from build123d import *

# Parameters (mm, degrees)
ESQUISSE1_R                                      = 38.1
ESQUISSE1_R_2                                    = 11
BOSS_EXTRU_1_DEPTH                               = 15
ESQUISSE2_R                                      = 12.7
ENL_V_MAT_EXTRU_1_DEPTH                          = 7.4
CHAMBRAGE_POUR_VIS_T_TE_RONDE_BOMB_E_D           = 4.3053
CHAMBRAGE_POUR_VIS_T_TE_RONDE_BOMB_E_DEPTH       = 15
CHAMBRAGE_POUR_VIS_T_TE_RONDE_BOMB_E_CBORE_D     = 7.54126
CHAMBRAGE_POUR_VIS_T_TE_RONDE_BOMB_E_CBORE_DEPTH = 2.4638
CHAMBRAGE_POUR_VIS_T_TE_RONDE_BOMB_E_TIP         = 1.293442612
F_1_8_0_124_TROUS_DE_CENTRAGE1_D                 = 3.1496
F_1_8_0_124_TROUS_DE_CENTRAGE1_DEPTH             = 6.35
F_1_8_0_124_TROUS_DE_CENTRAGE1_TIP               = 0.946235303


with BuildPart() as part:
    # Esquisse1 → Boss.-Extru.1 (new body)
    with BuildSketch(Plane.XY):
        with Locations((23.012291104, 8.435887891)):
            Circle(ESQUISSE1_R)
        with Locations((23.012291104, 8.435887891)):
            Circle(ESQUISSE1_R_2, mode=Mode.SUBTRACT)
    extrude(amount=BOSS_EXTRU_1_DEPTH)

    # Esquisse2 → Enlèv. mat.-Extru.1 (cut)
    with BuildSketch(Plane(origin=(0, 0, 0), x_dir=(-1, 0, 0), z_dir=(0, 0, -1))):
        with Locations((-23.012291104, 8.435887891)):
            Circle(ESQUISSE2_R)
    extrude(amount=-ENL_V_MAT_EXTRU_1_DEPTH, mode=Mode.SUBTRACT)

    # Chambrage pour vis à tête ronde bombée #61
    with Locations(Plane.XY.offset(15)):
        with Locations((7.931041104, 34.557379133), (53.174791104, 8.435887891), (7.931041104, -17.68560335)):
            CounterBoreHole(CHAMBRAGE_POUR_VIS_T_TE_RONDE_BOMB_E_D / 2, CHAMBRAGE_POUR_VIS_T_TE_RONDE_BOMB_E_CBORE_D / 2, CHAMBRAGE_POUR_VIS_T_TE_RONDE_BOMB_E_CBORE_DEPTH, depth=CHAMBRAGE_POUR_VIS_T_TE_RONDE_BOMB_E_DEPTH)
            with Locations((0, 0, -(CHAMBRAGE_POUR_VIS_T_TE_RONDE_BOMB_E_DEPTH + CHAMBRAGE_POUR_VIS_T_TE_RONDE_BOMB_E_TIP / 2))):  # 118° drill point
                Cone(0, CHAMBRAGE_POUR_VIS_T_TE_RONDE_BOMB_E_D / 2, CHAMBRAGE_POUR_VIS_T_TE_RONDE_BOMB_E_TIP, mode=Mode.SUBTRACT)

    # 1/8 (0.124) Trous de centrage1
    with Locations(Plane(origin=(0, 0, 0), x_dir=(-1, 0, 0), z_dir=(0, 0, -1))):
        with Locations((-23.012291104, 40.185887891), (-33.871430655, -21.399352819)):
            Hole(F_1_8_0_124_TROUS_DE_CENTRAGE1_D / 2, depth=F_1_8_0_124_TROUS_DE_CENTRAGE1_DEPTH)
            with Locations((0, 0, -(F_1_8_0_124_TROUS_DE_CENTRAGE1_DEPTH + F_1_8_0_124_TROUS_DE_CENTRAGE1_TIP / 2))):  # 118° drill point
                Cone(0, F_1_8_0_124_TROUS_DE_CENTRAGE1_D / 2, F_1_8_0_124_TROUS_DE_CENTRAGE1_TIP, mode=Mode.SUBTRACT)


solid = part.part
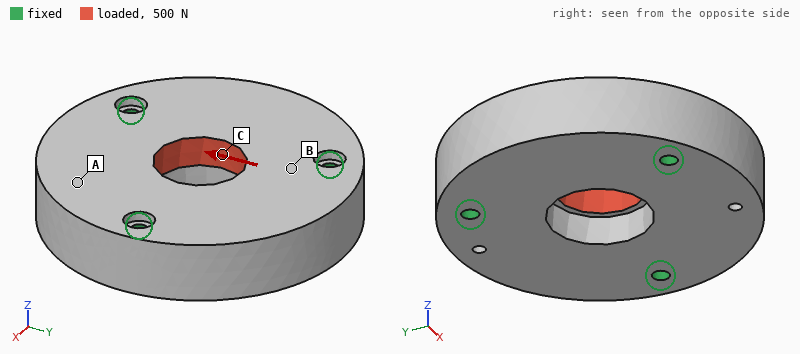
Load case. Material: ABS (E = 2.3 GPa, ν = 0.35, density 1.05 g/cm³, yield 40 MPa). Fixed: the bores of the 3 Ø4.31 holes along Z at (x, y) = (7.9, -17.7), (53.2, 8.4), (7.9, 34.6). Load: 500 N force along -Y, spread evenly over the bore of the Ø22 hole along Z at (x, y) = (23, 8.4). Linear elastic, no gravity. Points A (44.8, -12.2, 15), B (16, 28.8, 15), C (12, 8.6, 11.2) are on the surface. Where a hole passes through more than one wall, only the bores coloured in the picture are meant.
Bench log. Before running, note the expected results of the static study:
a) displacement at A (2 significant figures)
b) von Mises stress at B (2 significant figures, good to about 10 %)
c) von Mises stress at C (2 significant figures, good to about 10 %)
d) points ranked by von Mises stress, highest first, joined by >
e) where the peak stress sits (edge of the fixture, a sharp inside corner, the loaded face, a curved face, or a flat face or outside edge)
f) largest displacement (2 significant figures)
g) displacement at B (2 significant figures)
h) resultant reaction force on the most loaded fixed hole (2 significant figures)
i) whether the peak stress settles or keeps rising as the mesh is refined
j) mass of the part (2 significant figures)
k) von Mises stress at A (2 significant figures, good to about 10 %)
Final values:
10 µm
0.92 MPa
1.5 MPa
C > B > A
edge of the fixture
15 µm
6.8 µm
170 N
keeps rising
64 g
0.32 MPa
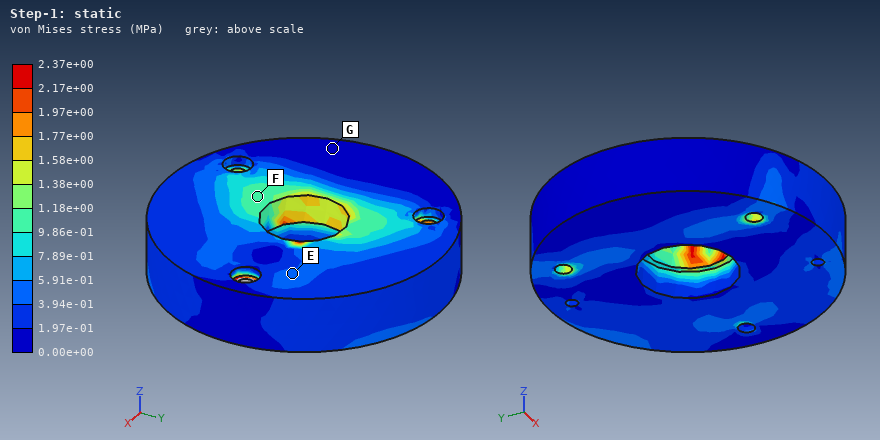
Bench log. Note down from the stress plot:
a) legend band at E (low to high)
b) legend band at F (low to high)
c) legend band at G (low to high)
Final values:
3.94e-01 to 5.91e-01 MPa
9.86e-01 to 1.18e+00 MPa
0.00e+00 to 1.97e-01 MPa
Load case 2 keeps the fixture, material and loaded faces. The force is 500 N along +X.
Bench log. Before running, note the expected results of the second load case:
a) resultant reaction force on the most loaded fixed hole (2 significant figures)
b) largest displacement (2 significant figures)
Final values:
170 N
17 µm
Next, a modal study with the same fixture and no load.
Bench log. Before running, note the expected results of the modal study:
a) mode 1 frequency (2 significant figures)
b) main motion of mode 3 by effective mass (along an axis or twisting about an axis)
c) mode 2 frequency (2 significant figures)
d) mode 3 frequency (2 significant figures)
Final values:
3300 Hz
along Z
3300 Hz
4000 Hz
